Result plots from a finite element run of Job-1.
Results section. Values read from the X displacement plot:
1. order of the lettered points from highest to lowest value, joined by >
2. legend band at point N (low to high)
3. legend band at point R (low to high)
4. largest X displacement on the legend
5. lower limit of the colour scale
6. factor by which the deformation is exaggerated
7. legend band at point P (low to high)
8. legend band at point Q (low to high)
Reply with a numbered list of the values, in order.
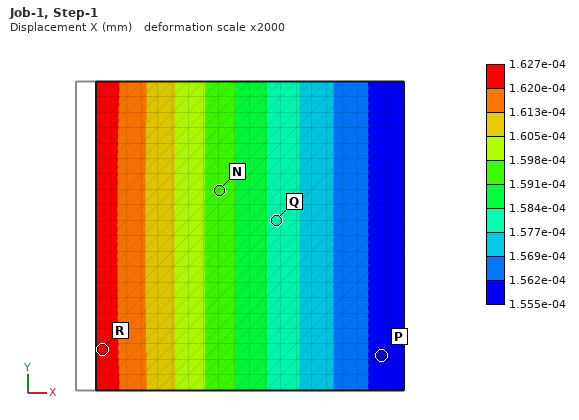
1. R > N > Q > P
2. 1.591e-04 to 1.598e-04 mm
3. 1.620e-04 to 1.627e-04 mm
4. 1.627e-04 mm
5. 1.555e-04 mm
6. 2000
7. 1.555e-04 to 1.562e-04 mm
8. 1.577e-04 to 1.584e-04 mm
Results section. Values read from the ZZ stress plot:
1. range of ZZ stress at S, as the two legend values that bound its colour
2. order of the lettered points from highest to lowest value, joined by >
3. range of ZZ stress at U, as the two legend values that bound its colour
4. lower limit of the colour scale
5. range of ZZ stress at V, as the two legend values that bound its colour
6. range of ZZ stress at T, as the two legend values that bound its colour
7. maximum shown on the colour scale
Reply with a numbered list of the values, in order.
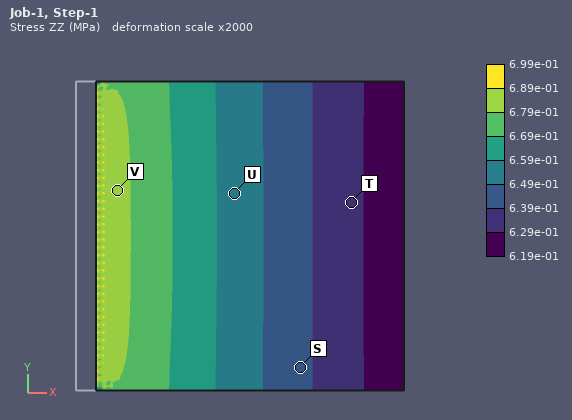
1. 6.39e-01 to 6.49e-01 MPa
2. V > U > S > T
3. 6.49e-01 to 6.59e-01 MPa
4. 6.19e-01 MPa
5. 6.79e-01 to 6.89e-01 MPa
6. 6.29e-01 to 6.39e-01 MPa
7. 6.99e-01 MPa
